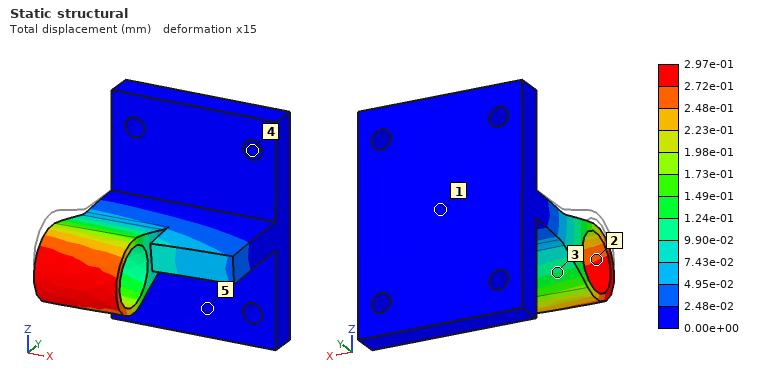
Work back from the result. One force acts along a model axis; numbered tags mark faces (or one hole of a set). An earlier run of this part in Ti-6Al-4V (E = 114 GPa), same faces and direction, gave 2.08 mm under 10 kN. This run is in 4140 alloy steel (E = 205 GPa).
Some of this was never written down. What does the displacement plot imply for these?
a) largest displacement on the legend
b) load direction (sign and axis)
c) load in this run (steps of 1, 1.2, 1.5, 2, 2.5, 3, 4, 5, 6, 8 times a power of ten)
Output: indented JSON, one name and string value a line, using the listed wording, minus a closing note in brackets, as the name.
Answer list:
{
  "largest displacement on the legend": "2.97e-01 mm",
  "load direction": "-Z",
  "load in this run": "2.5 kN"
}
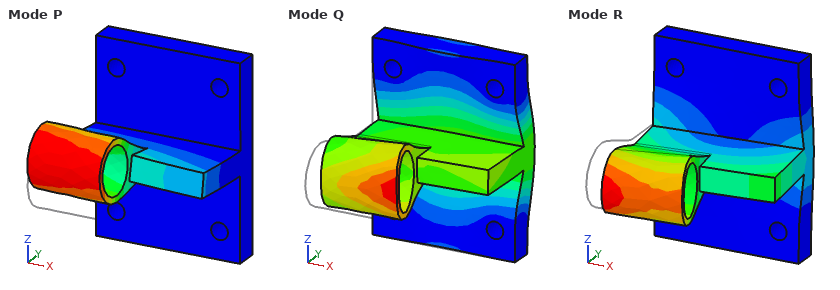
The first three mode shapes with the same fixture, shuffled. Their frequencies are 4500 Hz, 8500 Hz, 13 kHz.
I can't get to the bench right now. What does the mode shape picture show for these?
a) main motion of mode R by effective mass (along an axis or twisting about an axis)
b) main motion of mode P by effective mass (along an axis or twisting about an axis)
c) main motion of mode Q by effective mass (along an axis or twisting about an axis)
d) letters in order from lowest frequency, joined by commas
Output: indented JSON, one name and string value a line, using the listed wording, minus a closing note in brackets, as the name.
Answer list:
{
  "main motion of mode R by effective mass": "along X",
  "main motion of mode P by effective mass": "along Z",
  "main motion of mode Q by effective mass": "along Y",
  "letters in order from lowest frequency, joined by commas": "P, R, Q"
}
